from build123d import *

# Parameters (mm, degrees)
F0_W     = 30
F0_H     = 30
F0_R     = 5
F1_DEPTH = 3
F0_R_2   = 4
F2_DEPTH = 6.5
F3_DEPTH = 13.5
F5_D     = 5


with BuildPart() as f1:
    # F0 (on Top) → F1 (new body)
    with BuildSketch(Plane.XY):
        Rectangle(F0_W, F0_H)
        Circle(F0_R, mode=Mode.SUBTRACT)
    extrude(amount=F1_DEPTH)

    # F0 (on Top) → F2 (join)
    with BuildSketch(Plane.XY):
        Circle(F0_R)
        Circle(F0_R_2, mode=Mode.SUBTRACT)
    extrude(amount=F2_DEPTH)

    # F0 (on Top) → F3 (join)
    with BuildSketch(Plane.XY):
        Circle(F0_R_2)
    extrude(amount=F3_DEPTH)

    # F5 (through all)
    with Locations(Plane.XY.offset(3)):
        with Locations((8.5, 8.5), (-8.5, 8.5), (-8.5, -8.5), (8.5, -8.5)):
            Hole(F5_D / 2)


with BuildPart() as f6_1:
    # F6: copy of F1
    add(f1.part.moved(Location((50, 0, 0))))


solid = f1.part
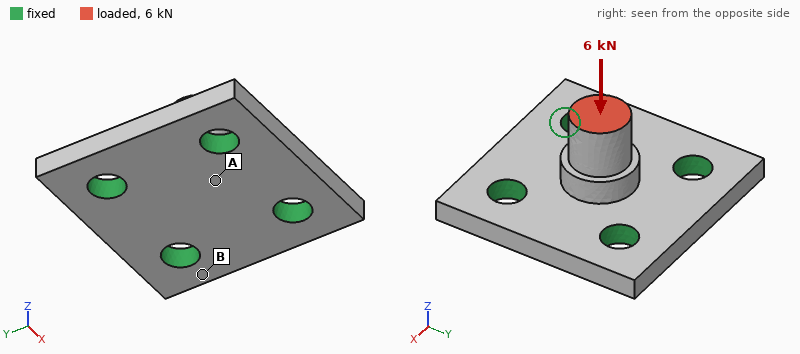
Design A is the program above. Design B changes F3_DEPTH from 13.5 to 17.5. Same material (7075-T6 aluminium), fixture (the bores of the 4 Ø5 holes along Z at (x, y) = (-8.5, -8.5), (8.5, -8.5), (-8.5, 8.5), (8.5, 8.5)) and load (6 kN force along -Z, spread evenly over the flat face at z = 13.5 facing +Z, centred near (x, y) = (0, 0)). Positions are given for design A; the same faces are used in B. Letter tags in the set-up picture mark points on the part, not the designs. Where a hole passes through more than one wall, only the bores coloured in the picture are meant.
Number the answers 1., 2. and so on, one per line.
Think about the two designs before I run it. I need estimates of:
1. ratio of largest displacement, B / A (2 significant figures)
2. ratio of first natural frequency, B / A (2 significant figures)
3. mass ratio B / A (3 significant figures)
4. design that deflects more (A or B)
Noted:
1. 1.1
2. 0.63
3. 1.07
4. B
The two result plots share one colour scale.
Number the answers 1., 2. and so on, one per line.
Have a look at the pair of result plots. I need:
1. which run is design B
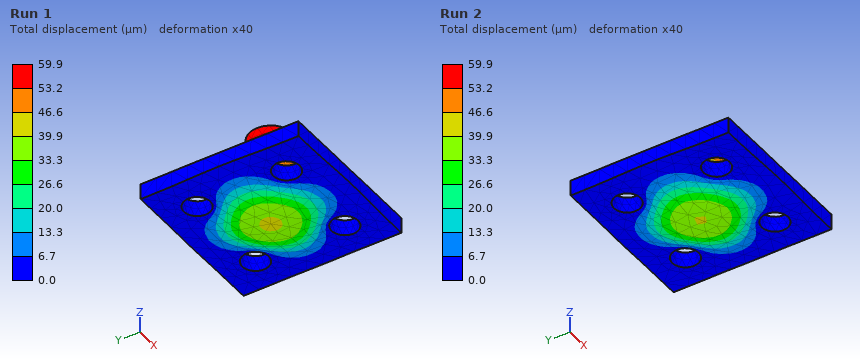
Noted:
1. Run 1
